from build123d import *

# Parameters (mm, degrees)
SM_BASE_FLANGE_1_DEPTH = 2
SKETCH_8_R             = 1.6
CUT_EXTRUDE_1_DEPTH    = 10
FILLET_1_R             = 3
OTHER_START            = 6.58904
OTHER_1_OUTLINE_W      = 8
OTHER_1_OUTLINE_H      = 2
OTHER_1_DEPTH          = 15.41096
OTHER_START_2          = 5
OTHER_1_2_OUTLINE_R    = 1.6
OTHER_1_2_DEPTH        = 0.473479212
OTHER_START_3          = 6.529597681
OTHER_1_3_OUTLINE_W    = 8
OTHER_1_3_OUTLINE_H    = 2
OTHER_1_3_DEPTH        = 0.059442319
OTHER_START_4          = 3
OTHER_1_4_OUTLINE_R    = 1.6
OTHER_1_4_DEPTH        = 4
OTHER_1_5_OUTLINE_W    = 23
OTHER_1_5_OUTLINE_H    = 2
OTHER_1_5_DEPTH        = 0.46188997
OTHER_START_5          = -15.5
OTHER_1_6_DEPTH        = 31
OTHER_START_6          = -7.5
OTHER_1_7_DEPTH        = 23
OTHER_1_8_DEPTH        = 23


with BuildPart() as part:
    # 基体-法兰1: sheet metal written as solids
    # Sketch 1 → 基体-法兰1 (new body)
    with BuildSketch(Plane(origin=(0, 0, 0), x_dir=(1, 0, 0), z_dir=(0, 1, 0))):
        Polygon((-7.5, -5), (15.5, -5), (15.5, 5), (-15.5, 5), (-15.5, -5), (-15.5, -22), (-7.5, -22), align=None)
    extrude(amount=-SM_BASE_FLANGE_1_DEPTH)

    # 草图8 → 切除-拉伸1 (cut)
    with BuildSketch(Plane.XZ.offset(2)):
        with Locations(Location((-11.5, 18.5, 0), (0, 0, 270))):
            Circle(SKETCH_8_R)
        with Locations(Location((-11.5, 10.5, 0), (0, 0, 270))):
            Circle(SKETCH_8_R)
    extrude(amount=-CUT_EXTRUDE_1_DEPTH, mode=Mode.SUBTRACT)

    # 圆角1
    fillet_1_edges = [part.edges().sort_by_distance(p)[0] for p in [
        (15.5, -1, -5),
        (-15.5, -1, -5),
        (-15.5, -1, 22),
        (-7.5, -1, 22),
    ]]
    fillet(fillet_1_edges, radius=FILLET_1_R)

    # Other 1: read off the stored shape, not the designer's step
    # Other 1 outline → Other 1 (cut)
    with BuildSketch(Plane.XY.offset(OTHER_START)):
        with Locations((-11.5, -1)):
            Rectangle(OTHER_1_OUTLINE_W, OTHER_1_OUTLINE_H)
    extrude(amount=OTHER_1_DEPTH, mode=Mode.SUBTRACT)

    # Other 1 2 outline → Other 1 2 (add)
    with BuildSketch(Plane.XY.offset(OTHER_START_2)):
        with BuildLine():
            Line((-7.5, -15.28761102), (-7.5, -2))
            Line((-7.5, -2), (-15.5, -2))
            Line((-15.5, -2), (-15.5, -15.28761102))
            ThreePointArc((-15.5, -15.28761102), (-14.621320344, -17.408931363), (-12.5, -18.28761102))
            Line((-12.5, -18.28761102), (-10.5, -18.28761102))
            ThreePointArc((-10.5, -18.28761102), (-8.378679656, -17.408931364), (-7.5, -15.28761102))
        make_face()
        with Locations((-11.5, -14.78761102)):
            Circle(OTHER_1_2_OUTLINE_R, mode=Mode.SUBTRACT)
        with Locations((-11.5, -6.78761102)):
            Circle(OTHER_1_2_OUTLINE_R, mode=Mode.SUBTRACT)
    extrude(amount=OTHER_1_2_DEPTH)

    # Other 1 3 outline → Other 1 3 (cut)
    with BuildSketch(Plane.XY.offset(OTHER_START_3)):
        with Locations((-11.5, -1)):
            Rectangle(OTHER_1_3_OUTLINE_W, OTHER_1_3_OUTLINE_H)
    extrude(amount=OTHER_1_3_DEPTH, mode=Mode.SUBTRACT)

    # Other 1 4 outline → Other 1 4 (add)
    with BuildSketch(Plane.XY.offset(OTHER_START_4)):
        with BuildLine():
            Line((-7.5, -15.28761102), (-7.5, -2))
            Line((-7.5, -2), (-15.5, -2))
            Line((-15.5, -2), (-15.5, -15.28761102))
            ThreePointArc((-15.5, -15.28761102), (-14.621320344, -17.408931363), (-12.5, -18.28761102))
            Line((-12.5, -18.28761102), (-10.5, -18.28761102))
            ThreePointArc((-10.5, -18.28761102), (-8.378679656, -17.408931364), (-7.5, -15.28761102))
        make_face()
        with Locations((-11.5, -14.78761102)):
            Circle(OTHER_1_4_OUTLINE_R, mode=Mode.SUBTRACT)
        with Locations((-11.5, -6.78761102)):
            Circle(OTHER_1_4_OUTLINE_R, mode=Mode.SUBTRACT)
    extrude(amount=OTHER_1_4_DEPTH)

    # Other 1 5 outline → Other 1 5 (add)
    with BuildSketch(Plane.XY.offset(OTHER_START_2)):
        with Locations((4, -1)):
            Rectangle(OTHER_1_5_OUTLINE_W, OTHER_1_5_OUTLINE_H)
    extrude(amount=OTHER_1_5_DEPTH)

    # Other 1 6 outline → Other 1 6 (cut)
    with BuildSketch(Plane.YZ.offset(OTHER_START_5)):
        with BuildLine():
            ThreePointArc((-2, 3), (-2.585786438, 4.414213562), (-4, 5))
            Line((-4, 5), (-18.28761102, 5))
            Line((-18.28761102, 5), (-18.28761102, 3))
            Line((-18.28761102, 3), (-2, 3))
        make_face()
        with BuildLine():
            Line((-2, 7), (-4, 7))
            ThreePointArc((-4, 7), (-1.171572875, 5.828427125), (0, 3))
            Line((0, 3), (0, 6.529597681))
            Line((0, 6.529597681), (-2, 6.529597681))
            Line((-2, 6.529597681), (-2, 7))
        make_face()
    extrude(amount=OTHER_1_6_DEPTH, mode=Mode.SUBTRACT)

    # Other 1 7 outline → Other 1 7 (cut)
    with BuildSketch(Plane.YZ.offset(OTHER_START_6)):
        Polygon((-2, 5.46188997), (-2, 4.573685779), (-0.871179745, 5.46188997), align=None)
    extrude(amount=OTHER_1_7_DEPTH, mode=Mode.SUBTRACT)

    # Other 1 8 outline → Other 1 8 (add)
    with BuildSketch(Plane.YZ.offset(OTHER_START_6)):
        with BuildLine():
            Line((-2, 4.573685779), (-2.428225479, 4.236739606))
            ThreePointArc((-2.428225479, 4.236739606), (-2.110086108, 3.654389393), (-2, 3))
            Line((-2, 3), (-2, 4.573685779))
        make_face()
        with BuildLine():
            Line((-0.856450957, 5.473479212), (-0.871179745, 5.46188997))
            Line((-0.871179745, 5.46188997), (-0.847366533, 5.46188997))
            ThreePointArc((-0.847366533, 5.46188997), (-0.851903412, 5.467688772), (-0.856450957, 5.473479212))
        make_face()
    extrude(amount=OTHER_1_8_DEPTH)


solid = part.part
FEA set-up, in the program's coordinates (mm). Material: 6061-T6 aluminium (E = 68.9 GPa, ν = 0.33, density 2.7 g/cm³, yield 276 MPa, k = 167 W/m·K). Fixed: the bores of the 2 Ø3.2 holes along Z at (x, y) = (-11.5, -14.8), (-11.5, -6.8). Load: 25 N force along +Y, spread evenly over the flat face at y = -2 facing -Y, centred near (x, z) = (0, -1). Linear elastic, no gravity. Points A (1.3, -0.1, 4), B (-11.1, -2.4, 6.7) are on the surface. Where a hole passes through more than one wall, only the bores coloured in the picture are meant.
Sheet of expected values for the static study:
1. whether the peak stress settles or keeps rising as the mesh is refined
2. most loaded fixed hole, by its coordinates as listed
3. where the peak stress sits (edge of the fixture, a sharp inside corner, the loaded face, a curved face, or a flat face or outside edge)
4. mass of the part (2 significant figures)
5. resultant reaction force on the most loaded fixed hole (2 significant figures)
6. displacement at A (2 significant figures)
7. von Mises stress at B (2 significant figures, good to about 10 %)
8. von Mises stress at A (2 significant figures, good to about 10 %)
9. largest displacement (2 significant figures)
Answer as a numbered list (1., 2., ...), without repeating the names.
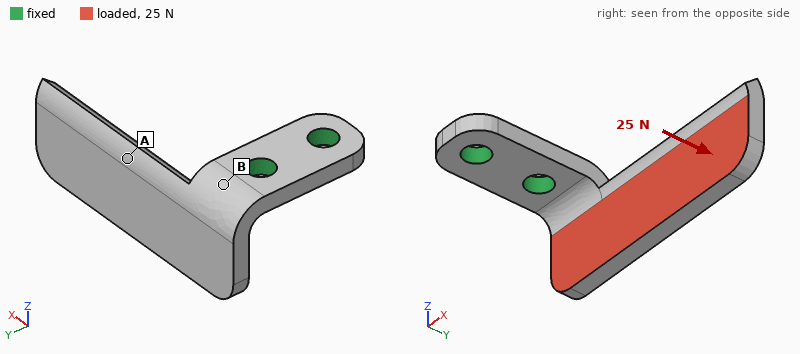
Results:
1. keeps rising
2. (-11.5, -6.8)
3. a sharp inside corner
4. 2.3 g
5. 26 N
6. 0.051 mm
7. 32 MPa
8. 12 MPa
9. 0.17 mm
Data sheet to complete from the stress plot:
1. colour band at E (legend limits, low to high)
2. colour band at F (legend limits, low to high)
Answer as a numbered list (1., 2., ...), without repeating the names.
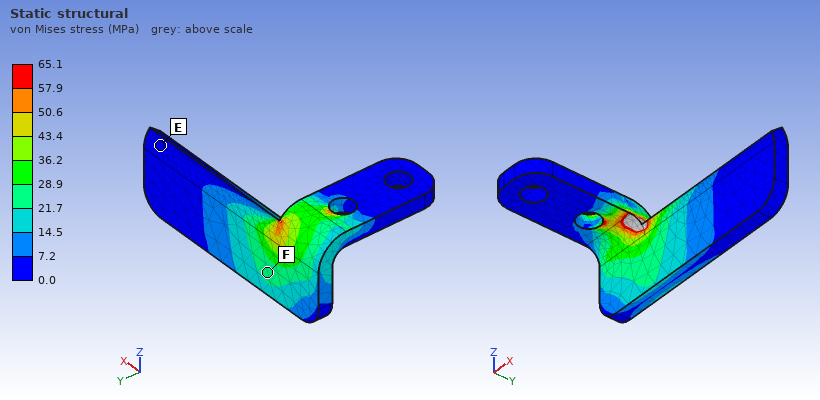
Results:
1. 0.0 to 7.2 MPa
2. 21.7 to 28.9 MPa
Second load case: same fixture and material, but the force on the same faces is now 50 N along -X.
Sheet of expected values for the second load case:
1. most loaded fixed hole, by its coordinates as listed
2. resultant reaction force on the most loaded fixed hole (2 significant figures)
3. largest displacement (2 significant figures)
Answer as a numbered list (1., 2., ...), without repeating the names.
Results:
1. (-11.5, -6.8)
2. 58 N
3. 83 µm
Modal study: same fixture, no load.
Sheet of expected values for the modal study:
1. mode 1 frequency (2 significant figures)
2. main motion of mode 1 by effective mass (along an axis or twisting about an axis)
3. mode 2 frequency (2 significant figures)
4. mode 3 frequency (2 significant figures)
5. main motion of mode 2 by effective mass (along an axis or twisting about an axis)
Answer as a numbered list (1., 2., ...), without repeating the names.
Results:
1. 1900 Hz
2. along Y
3. 3000 Hz
4. 5900 Hz
5. along Z
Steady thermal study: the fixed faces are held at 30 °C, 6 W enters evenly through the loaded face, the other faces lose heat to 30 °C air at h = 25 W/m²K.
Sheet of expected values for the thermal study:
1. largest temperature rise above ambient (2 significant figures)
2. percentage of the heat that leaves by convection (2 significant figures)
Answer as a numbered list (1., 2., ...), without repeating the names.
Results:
1. 33 K
2. 5.6 %
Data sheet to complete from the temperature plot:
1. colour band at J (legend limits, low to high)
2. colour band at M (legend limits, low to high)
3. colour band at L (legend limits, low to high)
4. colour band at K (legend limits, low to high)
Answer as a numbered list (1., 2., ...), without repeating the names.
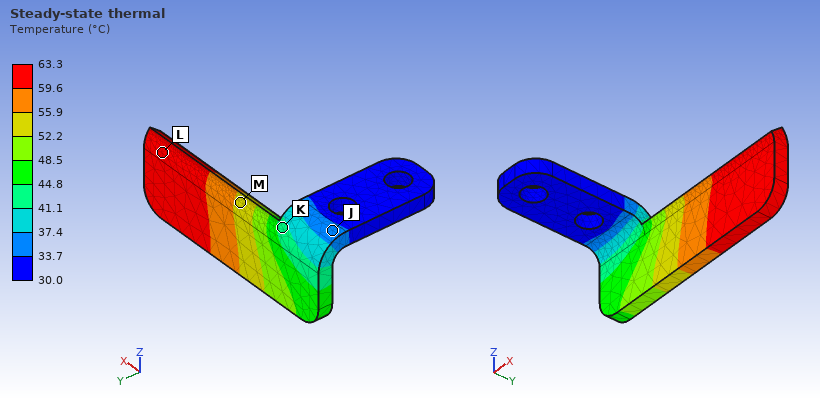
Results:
1. 33.7 to 37.4 °C
2. 52.2 to 55.9 °C
3. 59.6 to 63.3 °C
4. 41.1 to 44.8 °C
